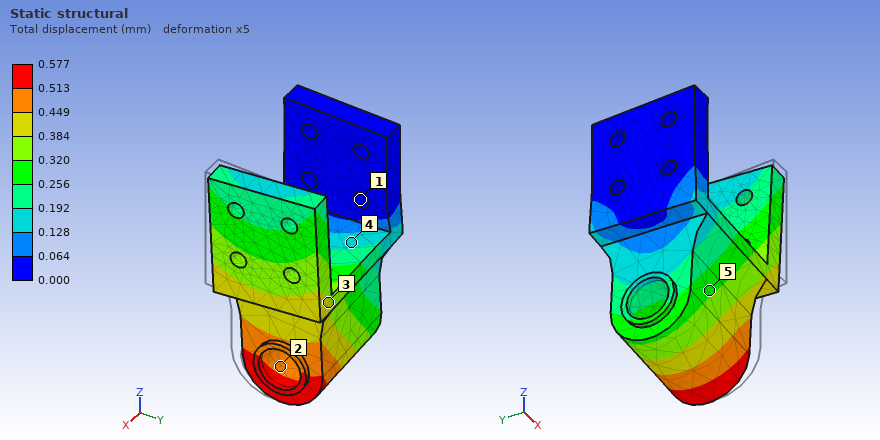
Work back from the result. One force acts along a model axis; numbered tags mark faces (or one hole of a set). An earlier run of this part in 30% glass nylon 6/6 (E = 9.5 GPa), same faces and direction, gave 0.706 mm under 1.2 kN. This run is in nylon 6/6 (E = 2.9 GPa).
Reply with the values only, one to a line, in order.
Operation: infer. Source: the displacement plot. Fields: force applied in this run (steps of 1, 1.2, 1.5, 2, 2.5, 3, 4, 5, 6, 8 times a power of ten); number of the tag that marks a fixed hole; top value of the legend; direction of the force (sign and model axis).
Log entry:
300 N
1
0.577 mm
+Y
